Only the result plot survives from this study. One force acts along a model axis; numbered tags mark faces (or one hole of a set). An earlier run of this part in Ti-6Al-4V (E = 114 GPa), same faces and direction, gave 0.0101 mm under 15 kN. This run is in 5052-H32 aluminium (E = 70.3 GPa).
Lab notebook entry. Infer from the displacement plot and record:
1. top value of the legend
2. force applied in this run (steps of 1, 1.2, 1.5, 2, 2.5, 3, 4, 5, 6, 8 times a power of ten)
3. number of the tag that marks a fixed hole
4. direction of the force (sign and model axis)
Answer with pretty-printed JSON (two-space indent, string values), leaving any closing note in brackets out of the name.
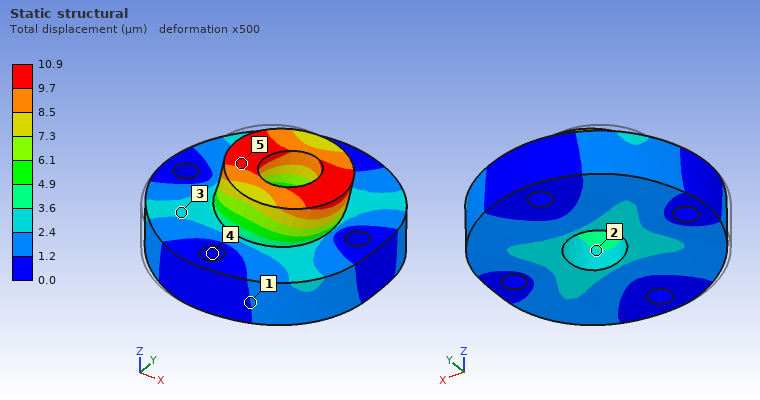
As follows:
{
  "top value of the legend": "10.9 µm",
  "force applied in this run": "10 kN",
  "number of the tag that marks a fixed hole": "4",
  "direction of the force": "+X"
}
